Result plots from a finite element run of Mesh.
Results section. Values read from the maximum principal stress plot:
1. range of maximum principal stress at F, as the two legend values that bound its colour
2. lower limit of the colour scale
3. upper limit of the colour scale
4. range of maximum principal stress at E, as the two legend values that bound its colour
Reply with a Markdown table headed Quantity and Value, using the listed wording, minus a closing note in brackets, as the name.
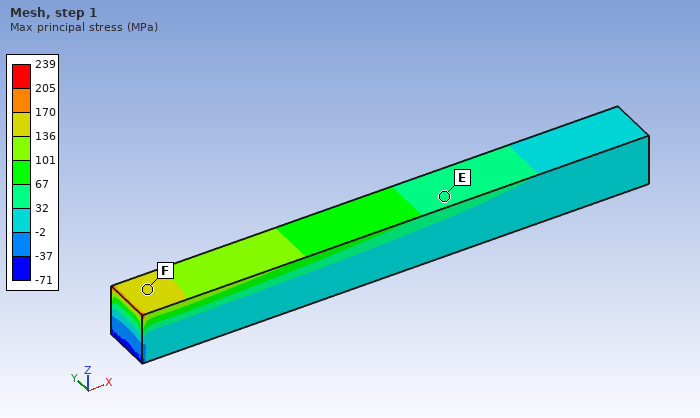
| Quantity | Value |
|---|---|
| range of maximum principal stress at F, as the two legend values that bound its colour | 136 to 170 MPa |
| lower limit of the colour scale | -71 MPa |
| upper limit of the colour scale | 239 MPa |
| range of maximum principal stress at E, as the two legend values that bound its colour | 32 to 67 MPa |
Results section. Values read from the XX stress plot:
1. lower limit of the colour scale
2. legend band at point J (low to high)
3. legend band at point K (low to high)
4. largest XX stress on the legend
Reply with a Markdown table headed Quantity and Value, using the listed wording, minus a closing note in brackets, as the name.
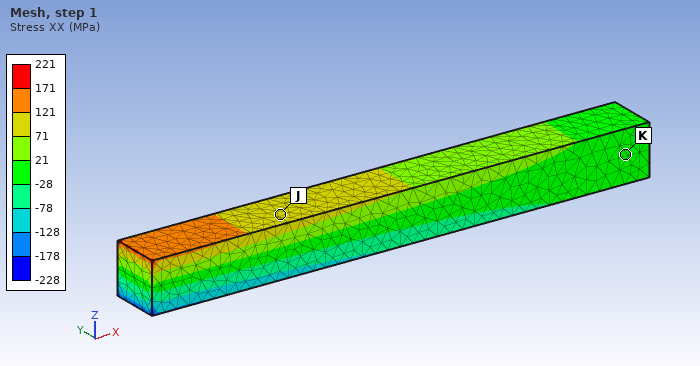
| Quantity | Value |
|---|---|
| lower limit of the colour scale | -228 MPa |
| legend band at point J | 71 to 121 MPa |
| legend band at point K | -28 to 21 MPa |
| largest XX stress on the legend | 221 MPa |
